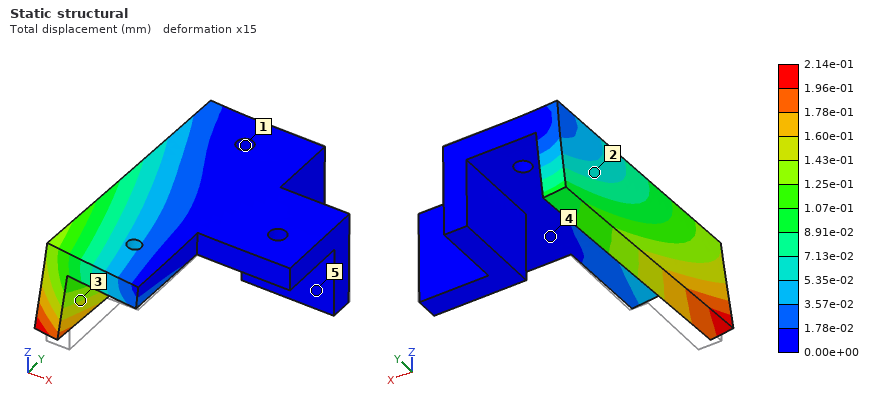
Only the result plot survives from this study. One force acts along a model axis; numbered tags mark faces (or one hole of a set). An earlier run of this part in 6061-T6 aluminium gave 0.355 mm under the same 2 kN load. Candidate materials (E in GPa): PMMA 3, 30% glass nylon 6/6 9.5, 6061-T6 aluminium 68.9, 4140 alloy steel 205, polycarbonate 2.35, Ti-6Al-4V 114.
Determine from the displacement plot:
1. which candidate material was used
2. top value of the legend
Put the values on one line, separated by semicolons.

Ti-6Al-4V; 2.14e-01 mm
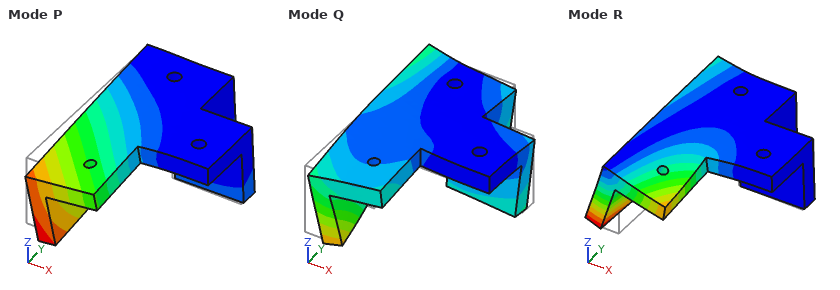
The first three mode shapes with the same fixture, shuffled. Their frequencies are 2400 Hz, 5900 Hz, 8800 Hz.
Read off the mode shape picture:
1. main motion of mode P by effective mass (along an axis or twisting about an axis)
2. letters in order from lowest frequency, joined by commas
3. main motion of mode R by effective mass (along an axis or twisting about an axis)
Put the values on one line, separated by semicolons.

along Z; P, R, Q; along X
